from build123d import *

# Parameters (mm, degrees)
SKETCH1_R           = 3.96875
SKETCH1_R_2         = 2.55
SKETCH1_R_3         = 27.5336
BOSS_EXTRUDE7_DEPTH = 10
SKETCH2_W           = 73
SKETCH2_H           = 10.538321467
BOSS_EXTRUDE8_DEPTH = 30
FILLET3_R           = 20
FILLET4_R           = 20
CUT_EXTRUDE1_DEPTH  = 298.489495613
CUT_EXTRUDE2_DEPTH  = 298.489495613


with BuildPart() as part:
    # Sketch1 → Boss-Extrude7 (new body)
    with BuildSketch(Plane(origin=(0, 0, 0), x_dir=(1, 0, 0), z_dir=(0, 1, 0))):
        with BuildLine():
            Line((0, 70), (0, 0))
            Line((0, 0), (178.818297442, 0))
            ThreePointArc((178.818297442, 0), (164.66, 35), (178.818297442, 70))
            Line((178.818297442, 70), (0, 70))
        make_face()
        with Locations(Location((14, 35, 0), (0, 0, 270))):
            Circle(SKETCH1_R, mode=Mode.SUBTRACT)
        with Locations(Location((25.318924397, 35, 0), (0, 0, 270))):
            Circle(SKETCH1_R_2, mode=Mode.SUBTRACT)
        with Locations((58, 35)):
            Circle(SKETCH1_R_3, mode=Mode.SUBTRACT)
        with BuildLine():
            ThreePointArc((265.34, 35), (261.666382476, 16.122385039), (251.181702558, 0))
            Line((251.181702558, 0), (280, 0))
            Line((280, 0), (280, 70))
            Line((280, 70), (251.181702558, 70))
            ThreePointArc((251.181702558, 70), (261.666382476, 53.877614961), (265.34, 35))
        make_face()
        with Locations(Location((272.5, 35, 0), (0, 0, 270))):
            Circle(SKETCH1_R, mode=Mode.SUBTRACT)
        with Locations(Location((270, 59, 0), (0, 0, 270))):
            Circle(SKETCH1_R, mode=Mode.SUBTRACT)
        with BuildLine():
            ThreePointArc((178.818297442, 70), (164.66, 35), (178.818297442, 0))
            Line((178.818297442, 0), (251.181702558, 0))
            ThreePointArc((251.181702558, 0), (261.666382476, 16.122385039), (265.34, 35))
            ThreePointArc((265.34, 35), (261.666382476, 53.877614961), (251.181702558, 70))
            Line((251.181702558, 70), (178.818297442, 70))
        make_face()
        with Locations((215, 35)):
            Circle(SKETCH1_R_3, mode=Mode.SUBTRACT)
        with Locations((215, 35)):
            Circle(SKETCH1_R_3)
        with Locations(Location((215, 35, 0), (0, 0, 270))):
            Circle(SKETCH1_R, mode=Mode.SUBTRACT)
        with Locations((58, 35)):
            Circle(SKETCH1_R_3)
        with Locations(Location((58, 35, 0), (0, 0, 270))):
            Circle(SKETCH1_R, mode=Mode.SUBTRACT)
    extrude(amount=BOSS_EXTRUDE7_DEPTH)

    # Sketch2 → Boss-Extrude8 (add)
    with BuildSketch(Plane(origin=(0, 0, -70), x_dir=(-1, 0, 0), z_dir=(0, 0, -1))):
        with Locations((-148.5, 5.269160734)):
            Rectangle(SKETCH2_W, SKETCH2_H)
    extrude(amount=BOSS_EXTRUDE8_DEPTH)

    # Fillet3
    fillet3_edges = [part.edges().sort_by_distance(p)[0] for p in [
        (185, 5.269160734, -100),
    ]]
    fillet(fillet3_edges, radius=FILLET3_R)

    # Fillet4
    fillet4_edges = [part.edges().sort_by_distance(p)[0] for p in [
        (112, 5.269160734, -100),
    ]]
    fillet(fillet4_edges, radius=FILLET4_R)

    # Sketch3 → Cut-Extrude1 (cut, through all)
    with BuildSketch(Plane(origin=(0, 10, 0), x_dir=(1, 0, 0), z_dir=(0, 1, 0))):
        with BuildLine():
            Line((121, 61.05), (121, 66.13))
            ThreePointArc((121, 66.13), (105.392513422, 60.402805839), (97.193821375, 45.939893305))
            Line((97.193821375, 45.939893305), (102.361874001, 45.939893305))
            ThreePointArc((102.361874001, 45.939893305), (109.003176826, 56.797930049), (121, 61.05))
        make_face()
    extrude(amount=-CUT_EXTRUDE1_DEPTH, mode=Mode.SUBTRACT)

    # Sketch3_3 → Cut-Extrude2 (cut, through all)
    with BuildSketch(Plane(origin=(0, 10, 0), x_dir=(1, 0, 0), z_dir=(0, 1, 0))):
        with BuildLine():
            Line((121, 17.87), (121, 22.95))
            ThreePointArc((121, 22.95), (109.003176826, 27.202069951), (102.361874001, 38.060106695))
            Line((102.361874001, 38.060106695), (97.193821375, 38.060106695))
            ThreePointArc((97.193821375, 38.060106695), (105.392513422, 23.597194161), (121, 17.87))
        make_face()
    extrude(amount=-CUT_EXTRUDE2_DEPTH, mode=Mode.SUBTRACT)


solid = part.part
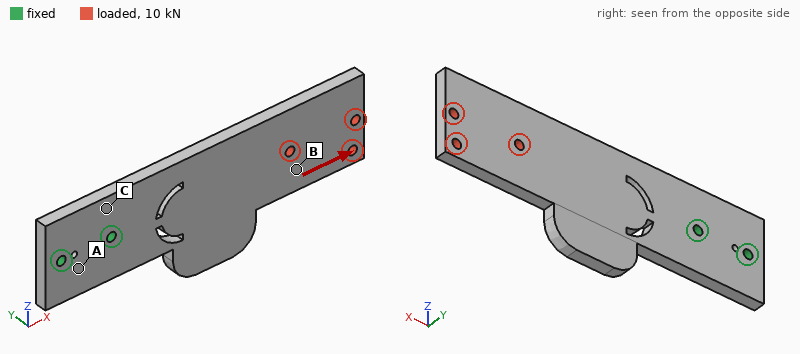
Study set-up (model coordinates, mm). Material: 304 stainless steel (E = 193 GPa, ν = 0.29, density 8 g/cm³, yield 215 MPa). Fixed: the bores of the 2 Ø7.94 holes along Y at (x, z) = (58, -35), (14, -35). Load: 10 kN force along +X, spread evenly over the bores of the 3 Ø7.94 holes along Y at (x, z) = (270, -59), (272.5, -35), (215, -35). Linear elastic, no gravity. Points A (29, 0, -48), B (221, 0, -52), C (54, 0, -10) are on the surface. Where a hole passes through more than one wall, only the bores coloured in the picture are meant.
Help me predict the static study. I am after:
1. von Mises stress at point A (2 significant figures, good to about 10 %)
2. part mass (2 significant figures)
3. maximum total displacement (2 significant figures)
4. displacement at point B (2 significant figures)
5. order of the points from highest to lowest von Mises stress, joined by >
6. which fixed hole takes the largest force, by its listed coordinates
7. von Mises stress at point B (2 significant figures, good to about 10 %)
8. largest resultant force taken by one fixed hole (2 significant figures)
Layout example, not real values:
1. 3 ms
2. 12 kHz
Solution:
1. 12 MPa
2. 1.7 kg
3. 59 µm
4. 38 µm
5. B > A > C
6. (58, -35)
7. 17 MPa
8. 7.9 kN
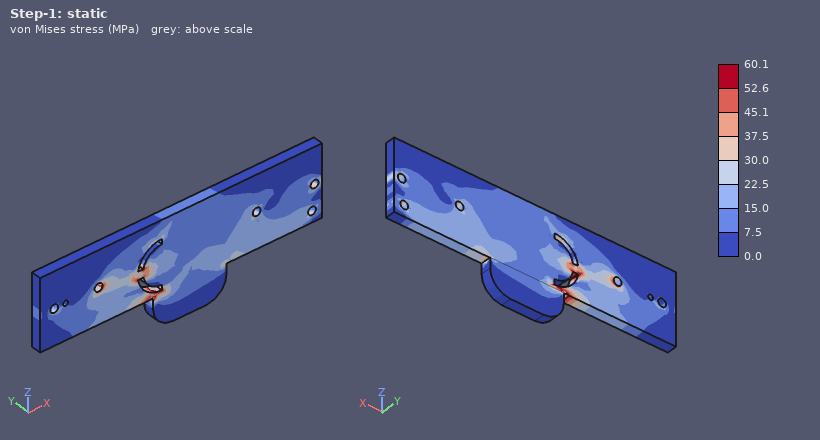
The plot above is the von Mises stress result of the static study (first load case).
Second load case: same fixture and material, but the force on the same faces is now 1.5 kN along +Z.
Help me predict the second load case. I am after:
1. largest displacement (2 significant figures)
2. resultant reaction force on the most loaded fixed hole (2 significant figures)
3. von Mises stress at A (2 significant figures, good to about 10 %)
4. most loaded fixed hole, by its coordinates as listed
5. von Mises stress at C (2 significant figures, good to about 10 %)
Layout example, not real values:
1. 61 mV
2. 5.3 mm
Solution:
1. 0.15 mm
2. 7.1 kN
3. 20 MPa
4. (58, -35)
5. 25 MPa
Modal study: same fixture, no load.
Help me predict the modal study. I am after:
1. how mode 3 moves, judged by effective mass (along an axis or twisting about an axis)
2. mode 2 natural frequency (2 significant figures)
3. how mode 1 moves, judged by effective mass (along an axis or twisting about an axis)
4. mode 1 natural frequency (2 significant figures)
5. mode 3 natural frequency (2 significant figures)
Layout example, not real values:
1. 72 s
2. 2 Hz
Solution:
1. along Z
2. 660 Hz
3. along Y
4. 150 Hz
5. 740 Hz
